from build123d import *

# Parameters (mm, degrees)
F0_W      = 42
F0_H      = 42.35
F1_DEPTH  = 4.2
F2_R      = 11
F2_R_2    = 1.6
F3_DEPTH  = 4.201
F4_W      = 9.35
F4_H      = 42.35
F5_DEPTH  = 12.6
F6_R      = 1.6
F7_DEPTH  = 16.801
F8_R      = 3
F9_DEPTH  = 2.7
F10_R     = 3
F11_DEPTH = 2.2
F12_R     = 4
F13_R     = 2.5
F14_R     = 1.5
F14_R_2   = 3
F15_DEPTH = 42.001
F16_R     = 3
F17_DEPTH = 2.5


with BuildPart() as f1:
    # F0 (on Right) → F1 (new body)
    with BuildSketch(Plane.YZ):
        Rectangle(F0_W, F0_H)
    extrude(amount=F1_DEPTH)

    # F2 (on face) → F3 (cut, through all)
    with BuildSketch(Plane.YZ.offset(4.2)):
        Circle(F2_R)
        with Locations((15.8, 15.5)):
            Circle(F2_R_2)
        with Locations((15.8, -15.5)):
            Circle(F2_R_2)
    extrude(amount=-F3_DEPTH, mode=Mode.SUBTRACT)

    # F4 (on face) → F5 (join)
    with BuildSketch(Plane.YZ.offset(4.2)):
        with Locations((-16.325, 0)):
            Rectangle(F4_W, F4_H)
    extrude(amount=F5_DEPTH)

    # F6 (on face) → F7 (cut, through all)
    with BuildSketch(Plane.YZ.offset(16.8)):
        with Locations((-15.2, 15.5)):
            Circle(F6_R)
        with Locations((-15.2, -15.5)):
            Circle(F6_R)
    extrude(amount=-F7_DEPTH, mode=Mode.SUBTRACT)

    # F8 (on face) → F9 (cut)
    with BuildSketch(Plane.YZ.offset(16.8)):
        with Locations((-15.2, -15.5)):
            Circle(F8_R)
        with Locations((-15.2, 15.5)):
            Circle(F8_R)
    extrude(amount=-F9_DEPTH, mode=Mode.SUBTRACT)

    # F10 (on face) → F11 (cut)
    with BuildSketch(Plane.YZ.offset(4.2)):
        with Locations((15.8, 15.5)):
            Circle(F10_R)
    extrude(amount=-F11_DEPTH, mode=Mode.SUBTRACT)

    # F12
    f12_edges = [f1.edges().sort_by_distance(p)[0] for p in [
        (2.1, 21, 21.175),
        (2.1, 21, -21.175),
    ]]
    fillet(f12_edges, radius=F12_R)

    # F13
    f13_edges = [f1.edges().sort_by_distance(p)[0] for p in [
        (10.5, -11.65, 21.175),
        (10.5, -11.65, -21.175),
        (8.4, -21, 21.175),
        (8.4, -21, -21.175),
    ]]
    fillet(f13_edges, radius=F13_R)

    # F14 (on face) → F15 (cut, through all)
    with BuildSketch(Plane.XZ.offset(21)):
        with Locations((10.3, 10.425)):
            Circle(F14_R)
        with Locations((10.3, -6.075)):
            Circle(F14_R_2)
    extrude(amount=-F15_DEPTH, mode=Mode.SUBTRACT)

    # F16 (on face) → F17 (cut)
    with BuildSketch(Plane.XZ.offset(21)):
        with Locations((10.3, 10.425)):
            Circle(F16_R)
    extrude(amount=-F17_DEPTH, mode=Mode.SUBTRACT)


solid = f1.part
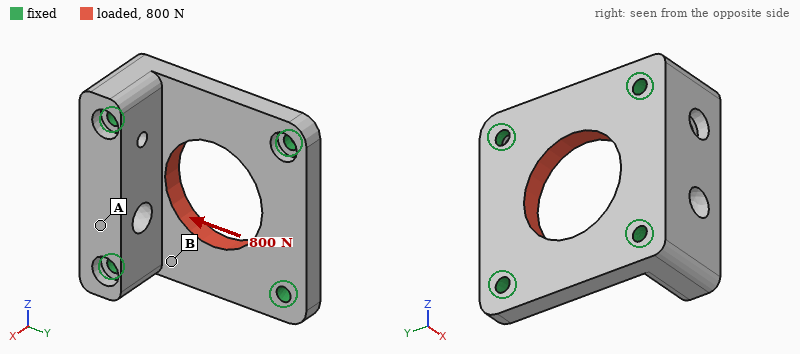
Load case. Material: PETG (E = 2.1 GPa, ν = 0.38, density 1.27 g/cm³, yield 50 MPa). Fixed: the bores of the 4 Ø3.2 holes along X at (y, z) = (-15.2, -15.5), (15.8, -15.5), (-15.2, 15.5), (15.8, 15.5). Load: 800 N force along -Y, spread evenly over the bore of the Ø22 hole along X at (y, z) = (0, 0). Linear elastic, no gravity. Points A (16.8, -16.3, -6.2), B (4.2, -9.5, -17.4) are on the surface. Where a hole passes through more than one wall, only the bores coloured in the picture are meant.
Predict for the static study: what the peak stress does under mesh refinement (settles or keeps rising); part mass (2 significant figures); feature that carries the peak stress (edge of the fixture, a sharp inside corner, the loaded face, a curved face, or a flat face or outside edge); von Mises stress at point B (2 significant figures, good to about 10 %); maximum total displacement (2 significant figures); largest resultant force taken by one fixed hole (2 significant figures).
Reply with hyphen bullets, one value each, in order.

- keeps rising
- 13 g
- edge of the fixture
- 3.2 MPa
- 74 µm
- 240 N
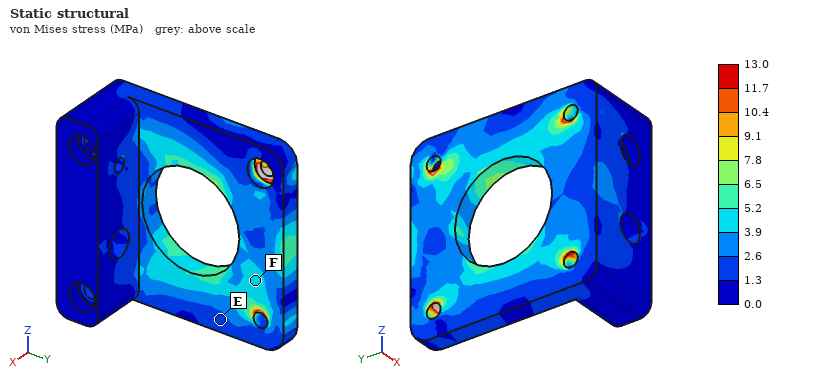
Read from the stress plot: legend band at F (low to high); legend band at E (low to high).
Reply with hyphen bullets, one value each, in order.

- 3.9 to 5.2 MPa
- 1.3 to 2.6 MPa
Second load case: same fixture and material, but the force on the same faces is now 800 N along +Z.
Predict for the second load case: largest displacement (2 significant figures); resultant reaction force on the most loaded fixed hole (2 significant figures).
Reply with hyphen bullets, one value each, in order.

- 65 µm
- 220 N
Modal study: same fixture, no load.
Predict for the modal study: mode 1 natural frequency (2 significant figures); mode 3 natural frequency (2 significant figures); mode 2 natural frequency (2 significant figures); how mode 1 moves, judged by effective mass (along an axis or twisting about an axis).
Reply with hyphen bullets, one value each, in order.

- 4800 Hz
- 6100 Hz
- 5200 Hz
- along X
